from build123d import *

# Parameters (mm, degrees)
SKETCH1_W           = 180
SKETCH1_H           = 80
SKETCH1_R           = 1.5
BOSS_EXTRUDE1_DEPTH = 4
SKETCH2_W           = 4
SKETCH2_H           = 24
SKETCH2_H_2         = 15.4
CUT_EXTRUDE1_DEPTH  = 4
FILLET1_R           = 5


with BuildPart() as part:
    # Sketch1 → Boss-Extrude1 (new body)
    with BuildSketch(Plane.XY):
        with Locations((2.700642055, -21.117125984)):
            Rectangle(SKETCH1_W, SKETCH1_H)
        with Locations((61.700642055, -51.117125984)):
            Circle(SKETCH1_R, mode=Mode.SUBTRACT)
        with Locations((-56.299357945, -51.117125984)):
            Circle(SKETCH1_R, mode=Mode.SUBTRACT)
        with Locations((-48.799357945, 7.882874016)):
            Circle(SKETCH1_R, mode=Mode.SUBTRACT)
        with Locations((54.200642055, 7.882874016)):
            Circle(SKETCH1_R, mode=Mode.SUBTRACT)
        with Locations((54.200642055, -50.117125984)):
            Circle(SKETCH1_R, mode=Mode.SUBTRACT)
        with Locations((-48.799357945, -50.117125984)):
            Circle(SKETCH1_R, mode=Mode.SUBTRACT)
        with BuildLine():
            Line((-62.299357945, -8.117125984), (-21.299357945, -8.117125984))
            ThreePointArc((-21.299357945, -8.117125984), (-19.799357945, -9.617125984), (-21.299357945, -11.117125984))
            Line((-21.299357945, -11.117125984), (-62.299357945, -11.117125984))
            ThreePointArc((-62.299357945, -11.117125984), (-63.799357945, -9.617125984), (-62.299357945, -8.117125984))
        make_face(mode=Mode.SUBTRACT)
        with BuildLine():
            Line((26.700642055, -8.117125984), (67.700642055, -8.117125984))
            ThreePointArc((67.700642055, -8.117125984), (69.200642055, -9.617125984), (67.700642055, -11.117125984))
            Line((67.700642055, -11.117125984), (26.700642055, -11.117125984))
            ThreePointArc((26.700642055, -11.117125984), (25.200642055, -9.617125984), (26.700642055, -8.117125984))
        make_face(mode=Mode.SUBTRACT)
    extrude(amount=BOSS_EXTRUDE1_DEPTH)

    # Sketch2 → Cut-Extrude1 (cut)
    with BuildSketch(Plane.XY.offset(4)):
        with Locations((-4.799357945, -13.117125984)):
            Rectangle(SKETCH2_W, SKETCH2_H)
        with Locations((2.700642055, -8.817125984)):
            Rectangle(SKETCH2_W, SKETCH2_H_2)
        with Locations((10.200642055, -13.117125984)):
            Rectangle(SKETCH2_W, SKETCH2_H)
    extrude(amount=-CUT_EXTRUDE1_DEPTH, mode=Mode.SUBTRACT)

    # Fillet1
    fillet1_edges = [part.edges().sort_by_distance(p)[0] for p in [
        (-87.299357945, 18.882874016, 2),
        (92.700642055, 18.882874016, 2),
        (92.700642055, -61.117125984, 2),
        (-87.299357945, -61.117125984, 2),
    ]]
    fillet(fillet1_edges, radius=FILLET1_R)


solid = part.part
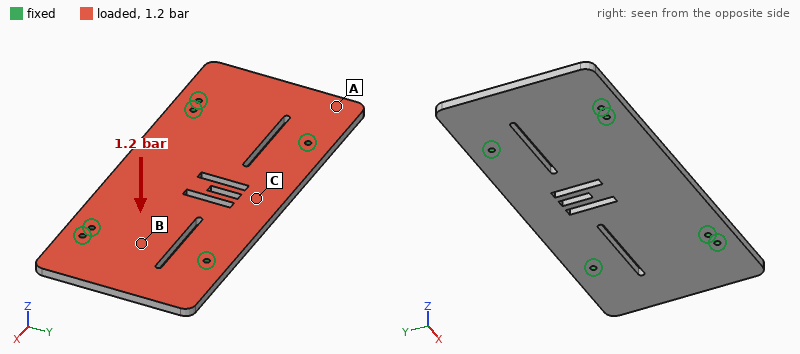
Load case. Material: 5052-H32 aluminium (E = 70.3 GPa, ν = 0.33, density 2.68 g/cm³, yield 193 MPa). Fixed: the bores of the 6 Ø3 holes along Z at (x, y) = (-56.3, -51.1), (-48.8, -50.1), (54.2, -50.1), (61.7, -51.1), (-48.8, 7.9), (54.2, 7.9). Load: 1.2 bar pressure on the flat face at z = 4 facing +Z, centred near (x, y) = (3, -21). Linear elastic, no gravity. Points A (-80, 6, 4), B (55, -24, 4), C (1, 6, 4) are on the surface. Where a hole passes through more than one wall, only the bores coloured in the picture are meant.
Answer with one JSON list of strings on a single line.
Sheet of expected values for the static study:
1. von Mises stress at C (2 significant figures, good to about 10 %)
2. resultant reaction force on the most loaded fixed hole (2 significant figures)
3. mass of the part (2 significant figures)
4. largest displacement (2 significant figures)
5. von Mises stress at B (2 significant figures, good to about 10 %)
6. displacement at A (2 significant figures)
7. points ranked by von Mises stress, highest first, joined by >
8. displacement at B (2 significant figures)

["26 MPa", "390 N", "150 g", "0.14 mm", "17 MPa", "0.057 mm", "C > B > A", "0.034 mm"]
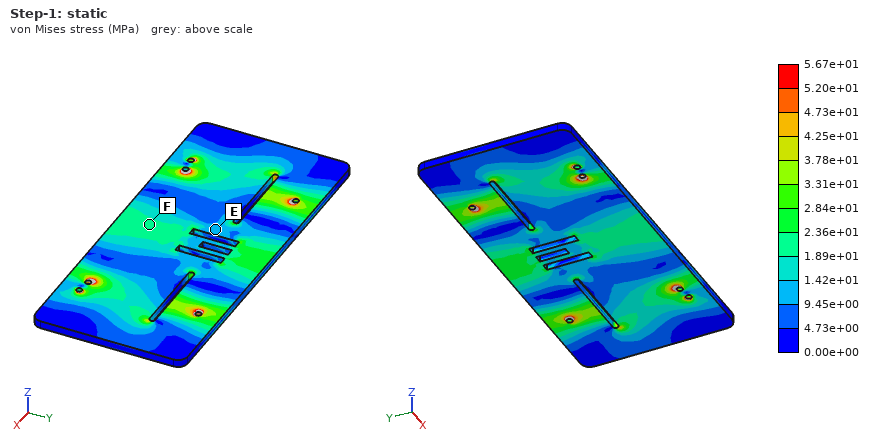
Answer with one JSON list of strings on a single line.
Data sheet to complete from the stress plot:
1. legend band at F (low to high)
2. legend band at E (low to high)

["1.89e+01 to 2.36e+01 MPa", "9.45e+00 to 1.42e+01 MPa"]
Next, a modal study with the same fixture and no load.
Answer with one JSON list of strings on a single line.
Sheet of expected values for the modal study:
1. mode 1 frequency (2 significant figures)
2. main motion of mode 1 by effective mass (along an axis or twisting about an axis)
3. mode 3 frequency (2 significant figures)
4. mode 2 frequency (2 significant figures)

["1600 Hz", "along Z", "2200 Hz", "2100 Hz"]
